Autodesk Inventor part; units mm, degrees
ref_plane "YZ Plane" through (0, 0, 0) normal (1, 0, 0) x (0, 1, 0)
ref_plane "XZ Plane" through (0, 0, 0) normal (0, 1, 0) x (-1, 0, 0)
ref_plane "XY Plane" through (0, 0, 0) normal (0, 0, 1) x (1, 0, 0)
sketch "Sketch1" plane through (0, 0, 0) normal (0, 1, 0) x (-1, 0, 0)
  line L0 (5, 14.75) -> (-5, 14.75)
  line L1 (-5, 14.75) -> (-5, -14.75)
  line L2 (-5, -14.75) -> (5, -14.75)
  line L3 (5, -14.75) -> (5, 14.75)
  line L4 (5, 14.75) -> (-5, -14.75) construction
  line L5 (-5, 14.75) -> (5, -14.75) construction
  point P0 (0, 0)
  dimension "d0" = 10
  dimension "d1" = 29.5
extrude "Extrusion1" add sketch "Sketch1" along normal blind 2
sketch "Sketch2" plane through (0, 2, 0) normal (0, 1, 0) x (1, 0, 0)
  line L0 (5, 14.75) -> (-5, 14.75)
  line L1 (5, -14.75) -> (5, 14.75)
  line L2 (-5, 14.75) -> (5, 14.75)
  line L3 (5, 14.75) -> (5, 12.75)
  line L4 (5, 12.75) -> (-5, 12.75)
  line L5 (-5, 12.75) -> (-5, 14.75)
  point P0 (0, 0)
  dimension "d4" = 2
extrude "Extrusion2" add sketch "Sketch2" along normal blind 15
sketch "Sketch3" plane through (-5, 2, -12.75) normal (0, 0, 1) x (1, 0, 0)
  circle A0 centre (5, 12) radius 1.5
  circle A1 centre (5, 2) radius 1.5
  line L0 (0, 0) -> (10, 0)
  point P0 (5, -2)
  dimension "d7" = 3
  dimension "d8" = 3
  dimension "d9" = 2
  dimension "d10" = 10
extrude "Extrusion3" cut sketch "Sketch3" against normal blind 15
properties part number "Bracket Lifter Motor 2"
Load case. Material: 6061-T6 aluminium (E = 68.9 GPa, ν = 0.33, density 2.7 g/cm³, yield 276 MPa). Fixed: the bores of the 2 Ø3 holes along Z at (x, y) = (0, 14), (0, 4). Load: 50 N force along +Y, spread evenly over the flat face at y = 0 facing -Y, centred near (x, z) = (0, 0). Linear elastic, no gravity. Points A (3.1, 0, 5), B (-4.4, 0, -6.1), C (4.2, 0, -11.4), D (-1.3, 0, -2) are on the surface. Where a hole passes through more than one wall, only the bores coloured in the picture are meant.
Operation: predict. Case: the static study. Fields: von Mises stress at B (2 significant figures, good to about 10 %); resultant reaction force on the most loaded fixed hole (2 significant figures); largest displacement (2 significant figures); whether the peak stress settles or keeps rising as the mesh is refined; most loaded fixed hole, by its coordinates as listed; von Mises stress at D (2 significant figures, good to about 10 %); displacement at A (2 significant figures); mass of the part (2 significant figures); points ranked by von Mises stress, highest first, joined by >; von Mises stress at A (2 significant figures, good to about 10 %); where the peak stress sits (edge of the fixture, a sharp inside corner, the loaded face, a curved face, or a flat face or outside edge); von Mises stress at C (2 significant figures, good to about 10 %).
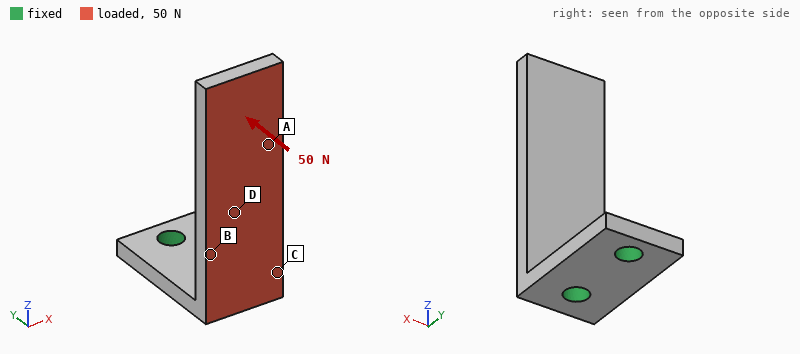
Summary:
56 MPa
54 N
0.37 mm
keeps rising
(0, 4)
36 MPa
0.21 mm
2.3 g
C > B > D > A
13 MPa
edge of the fixture
85 MPa
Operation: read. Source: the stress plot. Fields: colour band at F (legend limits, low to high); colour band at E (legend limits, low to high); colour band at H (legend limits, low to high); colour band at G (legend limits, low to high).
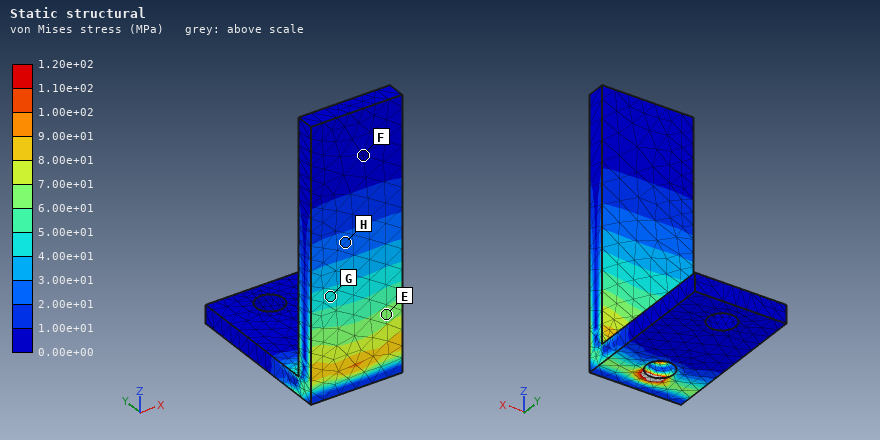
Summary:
0.00e+00 to 1.00e+01 MPa
6.00e+01 to 7.00e+01 MPa
2.00e+01 to 3.00e+01 MPa
4.00e+01 to 5.00e+01 MPa
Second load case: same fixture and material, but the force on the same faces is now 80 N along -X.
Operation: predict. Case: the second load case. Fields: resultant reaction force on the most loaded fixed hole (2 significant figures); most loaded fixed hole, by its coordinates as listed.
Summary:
93 N
(0, 4)
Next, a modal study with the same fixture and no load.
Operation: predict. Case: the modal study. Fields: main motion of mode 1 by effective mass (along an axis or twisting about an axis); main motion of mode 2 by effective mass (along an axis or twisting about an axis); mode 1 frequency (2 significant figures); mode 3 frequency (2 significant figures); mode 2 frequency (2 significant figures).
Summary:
along Y
along X
1800 Hz
11 kHz
4500 Hz
